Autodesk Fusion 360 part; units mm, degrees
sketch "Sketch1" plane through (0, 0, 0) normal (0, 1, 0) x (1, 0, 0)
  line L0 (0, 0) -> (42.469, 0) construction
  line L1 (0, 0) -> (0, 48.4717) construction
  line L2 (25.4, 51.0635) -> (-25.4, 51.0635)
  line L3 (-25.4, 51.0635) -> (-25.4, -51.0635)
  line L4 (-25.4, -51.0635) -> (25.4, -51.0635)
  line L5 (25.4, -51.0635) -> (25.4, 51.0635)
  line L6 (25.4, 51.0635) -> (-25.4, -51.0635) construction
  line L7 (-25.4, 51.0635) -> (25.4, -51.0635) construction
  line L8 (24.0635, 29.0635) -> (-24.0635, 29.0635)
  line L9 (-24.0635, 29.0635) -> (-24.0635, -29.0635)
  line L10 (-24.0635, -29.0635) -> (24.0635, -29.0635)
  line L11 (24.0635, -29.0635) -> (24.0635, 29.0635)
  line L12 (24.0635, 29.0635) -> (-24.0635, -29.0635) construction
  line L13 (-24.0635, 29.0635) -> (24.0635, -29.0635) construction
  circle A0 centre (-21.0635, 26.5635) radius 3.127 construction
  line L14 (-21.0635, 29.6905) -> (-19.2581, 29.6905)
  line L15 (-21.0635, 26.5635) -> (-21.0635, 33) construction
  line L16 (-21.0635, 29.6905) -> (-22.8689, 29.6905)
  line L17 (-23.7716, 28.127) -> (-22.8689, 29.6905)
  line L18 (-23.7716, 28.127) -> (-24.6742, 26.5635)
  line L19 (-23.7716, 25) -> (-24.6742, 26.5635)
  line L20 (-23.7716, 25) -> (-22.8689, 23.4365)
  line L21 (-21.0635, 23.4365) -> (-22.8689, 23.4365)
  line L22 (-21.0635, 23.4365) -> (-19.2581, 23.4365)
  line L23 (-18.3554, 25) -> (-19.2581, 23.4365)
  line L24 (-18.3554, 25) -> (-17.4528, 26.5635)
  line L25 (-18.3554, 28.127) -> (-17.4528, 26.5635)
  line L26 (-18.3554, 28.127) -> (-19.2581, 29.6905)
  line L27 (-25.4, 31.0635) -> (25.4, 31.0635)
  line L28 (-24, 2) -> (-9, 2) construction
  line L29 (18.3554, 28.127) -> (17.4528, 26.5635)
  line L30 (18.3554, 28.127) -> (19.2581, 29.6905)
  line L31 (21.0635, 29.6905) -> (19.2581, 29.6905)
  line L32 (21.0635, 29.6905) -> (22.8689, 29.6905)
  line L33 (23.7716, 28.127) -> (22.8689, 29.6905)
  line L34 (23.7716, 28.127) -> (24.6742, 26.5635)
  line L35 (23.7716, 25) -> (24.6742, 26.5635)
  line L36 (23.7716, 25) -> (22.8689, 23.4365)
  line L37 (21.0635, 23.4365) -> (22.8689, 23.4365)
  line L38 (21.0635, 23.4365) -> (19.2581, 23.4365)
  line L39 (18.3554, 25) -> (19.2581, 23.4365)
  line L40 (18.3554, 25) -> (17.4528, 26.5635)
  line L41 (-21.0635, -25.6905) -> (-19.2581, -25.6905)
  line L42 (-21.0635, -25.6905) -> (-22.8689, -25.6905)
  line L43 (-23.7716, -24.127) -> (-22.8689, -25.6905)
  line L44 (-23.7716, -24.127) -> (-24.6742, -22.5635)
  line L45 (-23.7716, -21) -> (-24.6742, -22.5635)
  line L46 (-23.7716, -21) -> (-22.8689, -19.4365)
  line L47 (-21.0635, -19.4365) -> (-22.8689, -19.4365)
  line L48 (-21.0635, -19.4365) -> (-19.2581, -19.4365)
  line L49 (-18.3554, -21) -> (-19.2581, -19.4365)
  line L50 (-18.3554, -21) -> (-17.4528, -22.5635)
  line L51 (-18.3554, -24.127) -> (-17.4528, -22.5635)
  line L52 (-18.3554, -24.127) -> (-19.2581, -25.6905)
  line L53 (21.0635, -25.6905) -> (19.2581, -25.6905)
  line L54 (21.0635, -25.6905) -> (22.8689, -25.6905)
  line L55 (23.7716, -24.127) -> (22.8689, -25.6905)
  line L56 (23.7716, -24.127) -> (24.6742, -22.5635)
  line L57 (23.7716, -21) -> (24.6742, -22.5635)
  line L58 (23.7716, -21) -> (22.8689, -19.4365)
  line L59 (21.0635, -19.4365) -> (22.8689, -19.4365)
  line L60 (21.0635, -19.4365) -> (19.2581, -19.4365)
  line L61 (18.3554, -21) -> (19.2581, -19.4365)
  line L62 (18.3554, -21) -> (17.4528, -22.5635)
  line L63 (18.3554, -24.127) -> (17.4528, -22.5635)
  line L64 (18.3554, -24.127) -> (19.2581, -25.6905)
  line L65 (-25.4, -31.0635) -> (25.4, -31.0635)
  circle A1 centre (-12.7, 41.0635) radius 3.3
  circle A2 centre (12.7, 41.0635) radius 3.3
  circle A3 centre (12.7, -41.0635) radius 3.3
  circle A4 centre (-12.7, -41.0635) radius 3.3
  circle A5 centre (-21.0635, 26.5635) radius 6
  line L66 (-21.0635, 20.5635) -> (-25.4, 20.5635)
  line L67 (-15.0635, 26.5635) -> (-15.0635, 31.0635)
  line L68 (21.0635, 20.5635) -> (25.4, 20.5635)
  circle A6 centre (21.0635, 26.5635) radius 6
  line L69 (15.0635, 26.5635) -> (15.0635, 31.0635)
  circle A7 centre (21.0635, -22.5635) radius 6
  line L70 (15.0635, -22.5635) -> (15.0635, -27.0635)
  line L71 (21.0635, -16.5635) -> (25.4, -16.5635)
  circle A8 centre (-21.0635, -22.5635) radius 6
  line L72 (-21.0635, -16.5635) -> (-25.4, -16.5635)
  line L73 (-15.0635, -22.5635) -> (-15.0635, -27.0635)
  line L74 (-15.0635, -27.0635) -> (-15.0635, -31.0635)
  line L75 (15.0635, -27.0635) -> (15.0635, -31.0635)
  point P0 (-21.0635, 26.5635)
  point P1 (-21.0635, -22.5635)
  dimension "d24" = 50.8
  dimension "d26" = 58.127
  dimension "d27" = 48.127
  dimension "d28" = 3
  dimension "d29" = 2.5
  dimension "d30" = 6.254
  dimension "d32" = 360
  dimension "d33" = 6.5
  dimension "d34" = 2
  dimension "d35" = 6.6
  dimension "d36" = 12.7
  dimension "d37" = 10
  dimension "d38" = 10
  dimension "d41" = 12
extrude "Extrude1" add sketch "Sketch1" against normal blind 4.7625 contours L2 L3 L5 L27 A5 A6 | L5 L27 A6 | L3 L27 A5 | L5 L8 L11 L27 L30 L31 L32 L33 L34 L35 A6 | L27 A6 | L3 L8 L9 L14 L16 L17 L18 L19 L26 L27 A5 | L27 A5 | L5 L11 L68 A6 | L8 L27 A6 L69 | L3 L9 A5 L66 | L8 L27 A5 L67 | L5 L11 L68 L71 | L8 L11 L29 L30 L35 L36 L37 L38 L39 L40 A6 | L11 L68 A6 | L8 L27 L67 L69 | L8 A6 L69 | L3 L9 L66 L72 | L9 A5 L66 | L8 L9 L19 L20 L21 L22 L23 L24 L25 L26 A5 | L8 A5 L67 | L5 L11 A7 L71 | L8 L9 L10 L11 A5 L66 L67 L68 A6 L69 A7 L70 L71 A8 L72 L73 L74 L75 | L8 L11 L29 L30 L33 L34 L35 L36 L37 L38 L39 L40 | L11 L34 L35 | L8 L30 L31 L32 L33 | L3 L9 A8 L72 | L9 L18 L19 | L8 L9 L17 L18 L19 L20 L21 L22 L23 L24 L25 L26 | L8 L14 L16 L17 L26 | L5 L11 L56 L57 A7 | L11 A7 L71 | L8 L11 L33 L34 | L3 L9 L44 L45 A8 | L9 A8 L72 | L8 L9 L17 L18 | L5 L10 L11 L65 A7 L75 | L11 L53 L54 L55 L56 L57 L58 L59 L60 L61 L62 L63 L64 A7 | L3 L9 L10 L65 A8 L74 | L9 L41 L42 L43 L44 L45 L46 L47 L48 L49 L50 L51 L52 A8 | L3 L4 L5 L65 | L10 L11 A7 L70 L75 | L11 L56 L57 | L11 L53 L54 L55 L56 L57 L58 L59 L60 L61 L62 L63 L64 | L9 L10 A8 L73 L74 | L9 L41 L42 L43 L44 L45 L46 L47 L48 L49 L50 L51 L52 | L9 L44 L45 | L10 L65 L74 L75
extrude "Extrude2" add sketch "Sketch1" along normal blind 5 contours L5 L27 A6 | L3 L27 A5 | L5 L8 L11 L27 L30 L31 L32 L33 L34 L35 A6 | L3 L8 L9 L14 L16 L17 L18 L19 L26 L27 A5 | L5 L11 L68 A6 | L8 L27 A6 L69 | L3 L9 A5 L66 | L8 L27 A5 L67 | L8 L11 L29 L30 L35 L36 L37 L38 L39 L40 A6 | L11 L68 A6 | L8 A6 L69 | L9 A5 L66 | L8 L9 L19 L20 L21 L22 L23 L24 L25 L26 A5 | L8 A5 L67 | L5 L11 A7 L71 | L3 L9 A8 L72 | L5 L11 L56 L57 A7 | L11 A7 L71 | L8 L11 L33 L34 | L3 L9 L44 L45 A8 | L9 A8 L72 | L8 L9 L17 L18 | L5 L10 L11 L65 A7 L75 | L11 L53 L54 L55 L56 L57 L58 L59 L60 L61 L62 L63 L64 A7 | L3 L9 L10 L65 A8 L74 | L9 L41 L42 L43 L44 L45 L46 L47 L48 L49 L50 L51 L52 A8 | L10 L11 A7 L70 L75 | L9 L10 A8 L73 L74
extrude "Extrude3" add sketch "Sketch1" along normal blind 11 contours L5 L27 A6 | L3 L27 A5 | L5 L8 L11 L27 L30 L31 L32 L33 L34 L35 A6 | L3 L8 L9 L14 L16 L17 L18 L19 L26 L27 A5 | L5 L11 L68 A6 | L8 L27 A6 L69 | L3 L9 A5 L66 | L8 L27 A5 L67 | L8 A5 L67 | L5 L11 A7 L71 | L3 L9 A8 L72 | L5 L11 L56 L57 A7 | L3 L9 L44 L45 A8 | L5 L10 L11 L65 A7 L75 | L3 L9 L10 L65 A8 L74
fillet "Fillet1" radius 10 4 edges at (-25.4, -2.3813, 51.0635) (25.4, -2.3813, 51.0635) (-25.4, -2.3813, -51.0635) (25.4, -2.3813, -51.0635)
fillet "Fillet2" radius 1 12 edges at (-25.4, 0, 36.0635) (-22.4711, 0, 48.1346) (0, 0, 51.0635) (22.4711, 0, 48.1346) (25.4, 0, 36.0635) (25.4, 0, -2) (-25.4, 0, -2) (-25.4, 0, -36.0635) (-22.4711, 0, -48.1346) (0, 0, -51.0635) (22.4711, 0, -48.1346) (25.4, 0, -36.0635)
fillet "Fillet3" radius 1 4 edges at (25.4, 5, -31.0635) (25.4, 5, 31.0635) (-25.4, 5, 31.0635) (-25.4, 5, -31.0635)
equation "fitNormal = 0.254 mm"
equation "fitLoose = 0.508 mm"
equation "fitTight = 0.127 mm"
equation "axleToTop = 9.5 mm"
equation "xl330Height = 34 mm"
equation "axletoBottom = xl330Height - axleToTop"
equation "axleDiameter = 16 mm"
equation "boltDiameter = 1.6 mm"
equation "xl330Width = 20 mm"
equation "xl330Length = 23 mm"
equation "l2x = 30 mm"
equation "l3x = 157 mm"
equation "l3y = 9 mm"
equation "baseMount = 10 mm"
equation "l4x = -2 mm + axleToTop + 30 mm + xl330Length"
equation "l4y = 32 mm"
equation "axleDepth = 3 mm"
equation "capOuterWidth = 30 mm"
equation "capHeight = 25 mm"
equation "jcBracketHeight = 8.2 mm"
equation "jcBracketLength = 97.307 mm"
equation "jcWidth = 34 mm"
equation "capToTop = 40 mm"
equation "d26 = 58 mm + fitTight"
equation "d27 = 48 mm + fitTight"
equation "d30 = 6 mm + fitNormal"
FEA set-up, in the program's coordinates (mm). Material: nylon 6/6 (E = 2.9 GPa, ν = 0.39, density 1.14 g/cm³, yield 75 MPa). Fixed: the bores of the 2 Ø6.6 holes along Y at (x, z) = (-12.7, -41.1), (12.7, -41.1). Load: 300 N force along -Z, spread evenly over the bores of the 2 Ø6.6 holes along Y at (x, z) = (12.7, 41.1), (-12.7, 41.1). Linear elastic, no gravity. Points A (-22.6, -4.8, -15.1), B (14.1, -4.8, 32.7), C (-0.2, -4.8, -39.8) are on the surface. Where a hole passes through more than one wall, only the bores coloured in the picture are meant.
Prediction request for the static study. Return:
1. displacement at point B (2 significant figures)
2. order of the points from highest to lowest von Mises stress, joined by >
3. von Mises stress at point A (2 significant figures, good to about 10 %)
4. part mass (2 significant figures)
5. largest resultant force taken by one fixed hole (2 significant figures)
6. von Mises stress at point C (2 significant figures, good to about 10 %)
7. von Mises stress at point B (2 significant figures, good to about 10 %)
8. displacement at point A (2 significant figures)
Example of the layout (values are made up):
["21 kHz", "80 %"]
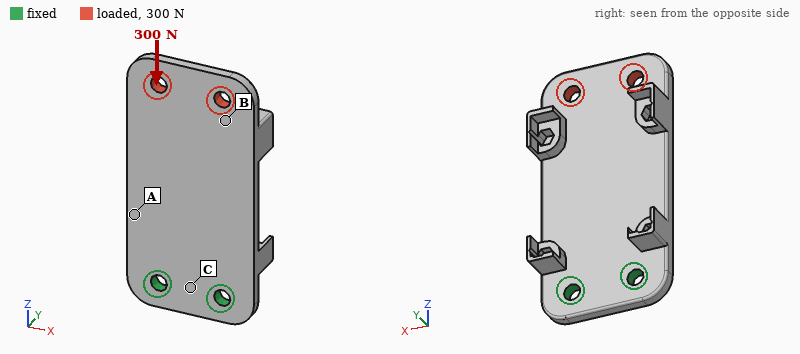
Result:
["38 µm", "B > A > C", "1.1 MPa", "30 g", "150 N", "0.48 MPa", "1.6 MPa", "14 µm"]
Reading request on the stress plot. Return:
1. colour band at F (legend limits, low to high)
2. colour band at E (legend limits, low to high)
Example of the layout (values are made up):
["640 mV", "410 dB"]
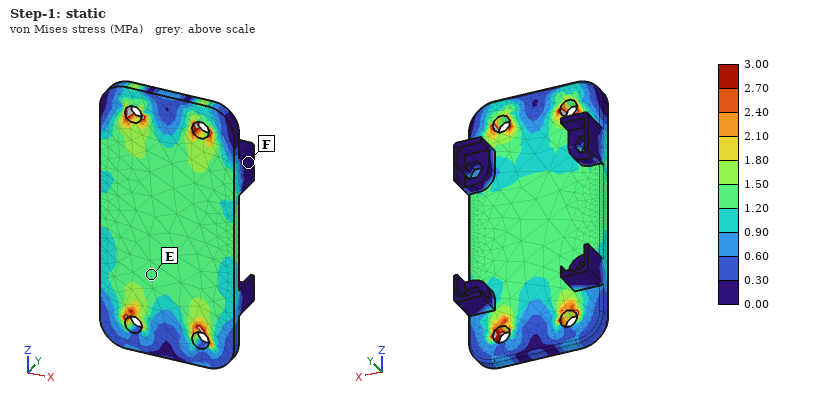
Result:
["0.00 to 0.30 MPa", "1.20 to 1.50 MPa"]
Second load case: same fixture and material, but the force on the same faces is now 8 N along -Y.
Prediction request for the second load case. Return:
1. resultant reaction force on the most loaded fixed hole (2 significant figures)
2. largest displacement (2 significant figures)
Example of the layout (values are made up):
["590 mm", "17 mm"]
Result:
["4.2 N", "1.1 mm"]
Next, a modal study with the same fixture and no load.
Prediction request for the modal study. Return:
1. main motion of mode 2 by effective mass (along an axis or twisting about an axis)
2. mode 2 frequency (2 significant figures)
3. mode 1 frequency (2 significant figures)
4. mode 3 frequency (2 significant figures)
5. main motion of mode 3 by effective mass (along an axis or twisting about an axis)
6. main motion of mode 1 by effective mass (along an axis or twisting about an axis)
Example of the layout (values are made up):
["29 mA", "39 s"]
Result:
["twisting about Z", "530 Hz", "160 Hz", "960 Hz", "along Y", "along Y"]
